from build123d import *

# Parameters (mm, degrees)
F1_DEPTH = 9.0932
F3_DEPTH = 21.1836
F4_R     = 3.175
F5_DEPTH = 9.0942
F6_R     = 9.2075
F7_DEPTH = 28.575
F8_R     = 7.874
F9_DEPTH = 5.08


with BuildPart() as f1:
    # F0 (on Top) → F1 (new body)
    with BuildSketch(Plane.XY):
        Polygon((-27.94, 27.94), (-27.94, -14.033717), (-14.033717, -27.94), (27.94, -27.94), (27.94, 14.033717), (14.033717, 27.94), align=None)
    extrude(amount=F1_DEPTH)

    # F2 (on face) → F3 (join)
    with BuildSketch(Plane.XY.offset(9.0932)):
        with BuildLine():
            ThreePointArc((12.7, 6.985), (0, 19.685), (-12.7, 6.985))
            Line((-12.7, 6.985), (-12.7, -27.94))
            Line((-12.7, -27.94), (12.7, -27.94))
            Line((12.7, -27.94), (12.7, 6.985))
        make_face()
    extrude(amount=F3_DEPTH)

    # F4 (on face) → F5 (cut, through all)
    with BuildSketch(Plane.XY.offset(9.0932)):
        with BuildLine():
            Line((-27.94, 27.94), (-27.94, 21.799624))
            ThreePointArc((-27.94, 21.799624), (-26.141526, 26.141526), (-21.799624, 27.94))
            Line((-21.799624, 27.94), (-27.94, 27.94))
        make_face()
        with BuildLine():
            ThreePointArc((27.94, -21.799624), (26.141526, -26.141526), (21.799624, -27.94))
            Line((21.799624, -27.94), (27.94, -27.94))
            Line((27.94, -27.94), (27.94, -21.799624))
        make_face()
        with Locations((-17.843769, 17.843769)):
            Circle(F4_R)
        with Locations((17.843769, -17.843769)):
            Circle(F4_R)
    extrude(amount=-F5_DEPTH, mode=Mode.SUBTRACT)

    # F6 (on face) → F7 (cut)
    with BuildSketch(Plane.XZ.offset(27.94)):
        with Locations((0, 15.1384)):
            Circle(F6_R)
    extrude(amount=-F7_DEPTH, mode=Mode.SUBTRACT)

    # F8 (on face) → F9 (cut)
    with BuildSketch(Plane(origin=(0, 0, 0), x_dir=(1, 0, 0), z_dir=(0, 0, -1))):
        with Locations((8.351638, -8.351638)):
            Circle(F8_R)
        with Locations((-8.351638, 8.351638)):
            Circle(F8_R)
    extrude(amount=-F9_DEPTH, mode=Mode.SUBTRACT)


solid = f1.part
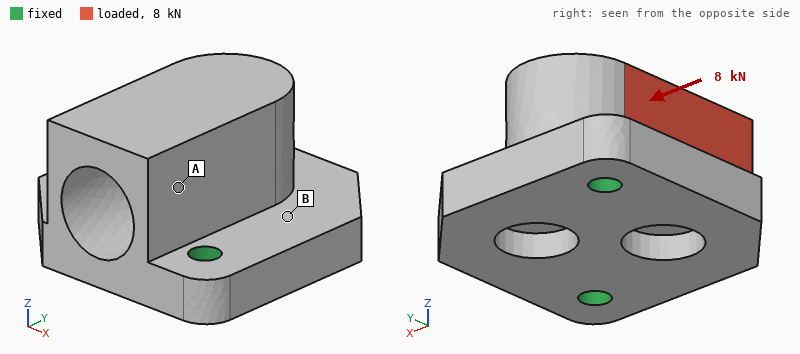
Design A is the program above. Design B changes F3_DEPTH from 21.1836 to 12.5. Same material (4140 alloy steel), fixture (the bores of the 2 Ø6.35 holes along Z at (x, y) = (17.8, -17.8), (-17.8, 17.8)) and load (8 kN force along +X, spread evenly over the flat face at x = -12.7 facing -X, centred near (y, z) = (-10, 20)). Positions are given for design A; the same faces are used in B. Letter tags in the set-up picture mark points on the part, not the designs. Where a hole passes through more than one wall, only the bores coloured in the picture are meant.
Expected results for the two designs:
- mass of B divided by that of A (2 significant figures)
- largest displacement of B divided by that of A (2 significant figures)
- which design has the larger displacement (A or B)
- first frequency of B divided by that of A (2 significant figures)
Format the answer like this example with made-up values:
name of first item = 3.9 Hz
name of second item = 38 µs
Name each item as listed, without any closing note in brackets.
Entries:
mass of B divided by that of A = 0.77
largest displacement of B divided by that of A = 2.3
which design has the larger displacement = B
first frequency of B divided by that of A = 1.3
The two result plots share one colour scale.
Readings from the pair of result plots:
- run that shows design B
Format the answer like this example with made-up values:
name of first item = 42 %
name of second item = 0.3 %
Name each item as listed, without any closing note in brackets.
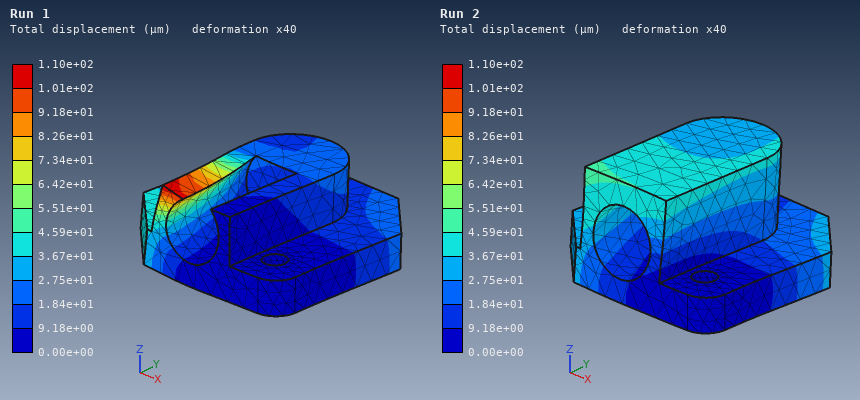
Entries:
run that shows design B = Run 1
